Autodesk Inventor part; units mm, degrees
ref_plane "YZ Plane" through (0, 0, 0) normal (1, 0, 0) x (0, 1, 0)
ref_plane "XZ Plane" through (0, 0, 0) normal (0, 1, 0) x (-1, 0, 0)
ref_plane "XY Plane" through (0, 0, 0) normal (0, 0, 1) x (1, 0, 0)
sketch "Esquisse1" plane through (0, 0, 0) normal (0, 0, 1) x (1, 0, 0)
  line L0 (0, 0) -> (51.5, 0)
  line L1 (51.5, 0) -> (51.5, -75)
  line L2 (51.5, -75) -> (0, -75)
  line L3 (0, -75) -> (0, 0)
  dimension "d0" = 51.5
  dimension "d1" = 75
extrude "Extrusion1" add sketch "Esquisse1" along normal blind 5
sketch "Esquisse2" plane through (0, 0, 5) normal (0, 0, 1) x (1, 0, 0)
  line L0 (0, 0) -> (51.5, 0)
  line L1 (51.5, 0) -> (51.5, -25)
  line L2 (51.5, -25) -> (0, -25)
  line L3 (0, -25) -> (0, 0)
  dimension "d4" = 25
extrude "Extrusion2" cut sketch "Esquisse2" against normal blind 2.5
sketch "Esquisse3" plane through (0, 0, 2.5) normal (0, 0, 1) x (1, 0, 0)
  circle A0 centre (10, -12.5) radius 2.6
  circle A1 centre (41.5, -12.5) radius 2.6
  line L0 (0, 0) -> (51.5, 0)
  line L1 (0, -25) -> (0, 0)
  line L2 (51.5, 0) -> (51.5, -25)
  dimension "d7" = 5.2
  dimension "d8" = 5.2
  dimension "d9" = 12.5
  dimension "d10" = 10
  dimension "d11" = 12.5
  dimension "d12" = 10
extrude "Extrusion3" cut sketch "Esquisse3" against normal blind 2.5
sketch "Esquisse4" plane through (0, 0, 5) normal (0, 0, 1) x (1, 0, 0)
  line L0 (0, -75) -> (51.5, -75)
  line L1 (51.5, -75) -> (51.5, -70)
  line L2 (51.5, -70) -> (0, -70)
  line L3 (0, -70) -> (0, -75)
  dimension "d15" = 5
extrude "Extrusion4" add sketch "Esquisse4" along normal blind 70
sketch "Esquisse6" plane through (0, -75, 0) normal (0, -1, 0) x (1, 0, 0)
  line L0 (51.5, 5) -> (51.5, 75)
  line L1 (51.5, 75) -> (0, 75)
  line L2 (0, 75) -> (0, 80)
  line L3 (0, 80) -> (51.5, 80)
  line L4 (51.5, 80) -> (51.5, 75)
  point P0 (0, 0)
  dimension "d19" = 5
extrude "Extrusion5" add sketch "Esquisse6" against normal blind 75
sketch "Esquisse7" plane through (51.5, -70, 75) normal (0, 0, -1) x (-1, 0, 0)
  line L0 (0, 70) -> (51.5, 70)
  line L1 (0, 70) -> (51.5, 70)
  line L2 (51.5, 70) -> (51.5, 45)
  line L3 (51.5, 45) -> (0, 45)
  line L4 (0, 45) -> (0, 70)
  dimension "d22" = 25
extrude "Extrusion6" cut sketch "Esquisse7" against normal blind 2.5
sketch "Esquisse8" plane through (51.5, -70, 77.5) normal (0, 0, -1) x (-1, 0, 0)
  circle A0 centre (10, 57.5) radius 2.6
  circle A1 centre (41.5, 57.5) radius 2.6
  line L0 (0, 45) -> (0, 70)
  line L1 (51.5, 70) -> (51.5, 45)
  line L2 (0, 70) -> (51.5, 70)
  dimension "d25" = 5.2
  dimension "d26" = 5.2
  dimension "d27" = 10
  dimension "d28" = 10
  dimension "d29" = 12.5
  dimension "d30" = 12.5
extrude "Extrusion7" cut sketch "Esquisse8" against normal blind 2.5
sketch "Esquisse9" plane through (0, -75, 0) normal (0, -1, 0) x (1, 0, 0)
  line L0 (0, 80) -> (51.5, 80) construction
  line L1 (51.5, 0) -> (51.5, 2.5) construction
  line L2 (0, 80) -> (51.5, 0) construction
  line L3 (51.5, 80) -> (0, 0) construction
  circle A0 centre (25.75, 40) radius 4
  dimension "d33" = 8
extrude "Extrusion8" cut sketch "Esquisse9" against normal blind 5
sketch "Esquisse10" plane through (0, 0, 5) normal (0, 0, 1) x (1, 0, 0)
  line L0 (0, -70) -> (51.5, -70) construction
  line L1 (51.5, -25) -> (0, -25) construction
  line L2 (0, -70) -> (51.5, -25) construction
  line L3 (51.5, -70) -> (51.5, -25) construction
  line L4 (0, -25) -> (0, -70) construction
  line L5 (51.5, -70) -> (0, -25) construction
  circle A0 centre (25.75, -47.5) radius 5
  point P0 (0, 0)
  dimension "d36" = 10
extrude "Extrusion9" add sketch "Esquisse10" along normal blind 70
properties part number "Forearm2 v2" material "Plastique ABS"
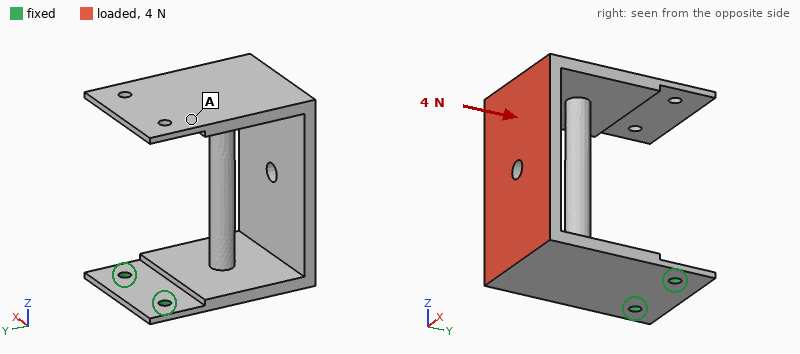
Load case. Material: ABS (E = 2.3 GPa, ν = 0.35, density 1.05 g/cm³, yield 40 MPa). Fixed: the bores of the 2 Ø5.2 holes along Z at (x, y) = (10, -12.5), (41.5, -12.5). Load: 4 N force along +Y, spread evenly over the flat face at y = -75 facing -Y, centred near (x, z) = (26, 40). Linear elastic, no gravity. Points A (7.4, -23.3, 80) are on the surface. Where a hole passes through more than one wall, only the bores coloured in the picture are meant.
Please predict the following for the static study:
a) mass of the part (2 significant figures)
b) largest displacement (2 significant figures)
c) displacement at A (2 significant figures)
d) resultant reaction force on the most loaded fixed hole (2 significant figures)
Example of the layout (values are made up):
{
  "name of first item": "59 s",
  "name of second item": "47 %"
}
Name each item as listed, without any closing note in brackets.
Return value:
{
  "mass of the part": "58 g",
  "largest displacement": "1.4 mm",
  "displacement at A": "1.2 mm",
  "resultant reaction force on the most loaded fixed hole": "2.0 N"
}
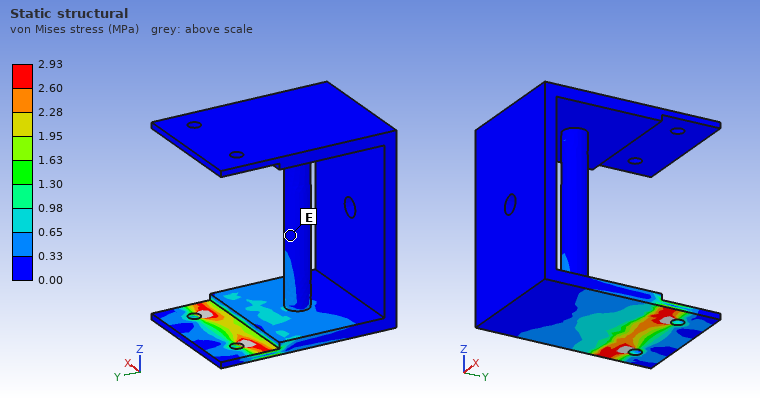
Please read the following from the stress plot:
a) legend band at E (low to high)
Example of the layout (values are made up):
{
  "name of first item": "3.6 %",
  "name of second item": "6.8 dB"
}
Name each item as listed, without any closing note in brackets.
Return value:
{
  "legend band at E": "0.00 to 0.33 MPa"
}
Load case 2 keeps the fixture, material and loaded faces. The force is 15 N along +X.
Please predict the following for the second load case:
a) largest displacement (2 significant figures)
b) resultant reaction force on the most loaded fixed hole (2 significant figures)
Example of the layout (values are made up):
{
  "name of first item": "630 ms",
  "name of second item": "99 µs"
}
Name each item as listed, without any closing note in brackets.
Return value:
{
  "largest displacement": "1.3 mm",
  "resultant reaction force on the most loaded fixed hole": "33 N"
}
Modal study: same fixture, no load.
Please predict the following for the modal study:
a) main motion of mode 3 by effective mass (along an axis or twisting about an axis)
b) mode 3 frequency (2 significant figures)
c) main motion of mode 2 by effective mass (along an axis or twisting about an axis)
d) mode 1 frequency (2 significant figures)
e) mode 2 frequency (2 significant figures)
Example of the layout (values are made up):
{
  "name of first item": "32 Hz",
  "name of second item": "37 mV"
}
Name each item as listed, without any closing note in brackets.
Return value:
{
  "main motion of mode 3 by effective mass": "along Z",
  "mode 3 frequency": "240 Hz",
  "main motion of mode 2 by effective mass": "along X",
  "mode 1 frequency": "34 Hz",
  "mode 2 frequency": "76 Hz"
}
